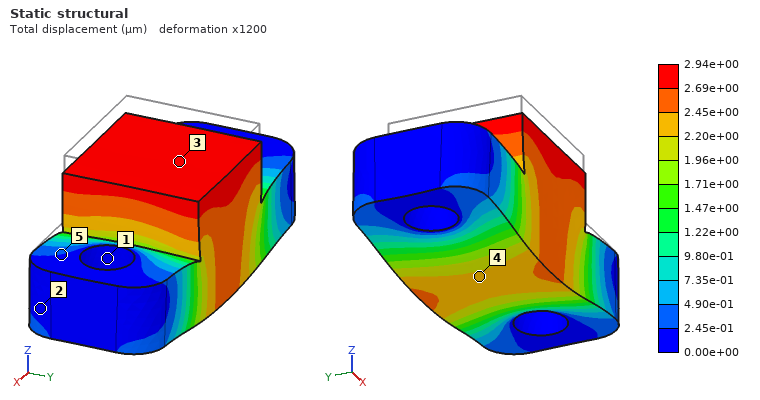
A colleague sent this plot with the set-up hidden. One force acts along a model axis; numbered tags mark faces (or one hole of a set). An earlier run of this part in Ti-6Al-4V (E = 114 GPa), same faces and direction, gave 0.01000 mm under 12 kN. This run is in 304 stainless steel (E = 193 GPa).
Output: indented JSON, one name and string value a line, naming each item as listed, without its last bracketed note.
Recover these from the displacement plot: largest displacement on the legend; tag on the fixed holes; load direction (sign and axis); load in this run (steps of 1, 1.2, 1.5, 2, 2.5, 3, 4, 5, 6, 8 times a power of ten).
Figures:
{
  "largest displacement on the legend": "2.94e+00 µm",
  "tag on the fixed holes": "1",
  "load direction": "-Z",
  "load in this run": "6 kN"
}
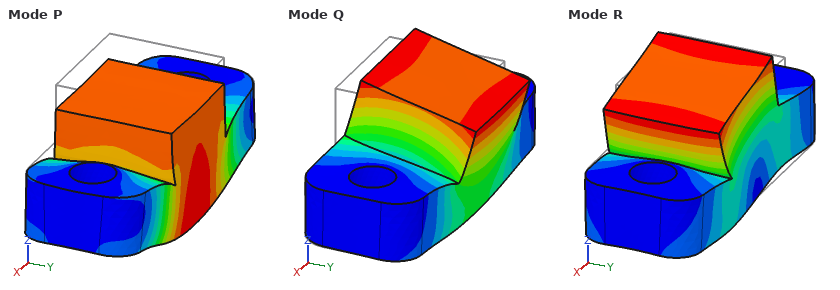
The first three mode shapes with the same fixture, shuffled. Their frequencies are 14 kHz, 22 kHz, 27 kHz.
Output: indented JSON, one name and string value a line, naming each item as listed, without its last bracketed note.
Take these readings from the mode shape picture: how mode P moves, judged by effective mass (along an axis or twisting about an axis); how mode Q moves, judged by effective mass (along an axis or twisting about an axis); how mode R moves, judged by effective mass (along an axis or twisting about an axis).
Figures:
{
  "how mode P moves, judged by effective mass": "along Z",
  "how mode Q moves, judged by effective mass": "along Y",
  "how mode R moves, judged by effective mass": "along X"
}
